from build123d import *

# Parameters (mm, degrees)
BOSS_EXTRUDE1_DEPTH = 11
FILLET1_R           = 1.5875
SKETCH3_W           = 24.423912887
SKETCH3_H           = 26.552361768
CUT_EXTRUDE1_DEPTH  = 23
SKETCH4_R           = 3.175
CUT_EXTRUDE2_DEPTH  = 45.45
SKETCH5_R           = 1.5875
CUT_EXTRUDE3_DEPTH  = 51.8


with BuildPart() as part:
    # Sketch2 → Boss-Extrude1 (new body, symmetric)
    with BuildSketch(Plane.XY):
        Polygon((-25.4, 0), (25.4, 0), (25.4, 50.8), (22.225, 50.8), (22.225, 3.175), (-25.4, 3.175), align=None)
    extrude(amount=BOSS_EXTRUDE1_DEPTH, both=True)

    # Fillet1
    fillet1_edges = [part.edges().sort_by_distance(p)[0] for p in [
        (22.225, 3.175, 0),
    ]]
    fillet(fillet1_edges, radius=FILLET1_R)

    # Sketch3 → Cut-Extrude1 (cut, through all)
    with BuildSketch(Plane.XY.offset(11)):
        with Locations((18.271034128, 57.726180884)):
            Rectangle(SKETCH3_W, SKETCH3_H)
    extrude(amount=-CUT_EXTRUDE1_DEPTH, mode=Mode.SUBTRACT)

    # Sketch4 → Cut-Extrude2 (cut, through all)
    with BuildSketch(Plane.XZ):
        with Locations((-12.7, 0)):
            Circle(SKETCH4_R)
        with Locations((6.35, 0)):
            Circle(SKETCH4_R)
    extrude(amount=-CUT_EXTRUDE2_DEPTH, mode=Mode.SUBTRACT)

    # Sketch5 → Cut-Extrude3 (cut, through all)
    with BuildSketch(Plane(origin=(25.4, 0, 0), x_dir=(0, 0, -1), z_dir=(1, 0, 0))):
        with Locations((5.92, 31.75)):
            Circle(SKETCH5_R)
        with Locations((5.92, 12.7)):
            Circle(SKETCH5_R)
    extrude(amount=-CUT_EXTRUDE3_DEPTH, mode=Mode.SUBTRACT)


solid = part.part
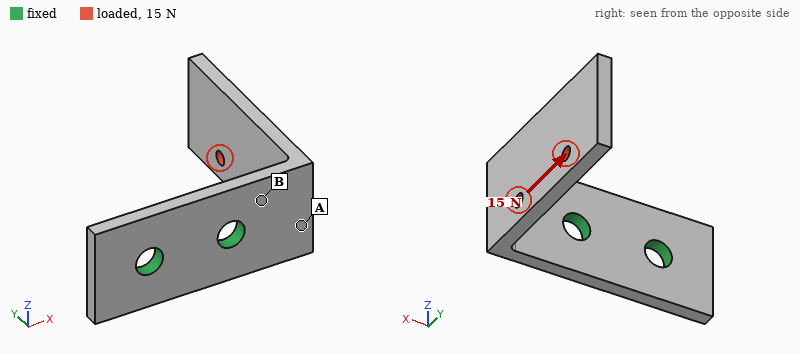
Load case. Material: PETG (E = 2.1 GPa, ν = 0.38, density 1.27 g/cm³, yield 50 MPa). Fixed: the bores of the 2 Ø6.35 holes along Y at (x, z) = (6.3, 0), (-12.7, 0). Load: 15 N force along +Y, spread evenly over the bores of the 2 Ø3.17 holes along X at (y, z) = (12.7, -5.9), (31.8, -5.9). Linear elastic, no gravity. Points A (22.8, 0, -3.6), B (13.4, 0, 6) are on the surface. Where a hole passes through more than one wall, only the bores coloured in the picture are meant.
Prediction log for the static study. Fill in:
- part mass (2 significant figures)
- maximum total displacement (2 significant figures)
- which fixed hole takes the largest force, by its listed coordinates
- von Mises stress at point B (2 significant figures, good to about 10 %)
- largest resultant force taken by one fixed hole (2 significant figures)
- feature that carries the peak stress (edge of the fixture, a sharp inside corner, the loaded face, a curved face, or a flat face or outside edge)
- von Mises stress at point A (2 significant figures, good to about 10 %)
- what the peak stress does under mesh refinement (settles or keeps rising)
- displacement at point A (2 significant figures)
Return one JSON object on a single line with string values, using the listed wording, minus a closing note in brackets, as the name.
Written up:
{"part mass": "7.9 g", "maximum total displacement": "0.72 mm", "which fixed hole takes the largest force, by its listed coordinates": "(6.3, 0)", "von Mises stress at point B": "3.6 MPa", "largest resultant force taken by one fixed hole": "16 N", "feature that carries the peak stress": "edge of the fixture", "von Mises stress at point A": "1.1 MPa", "what the peak stress does under mesh refinement": "keeps rising", "displacement at point A": "0.17 mm"}
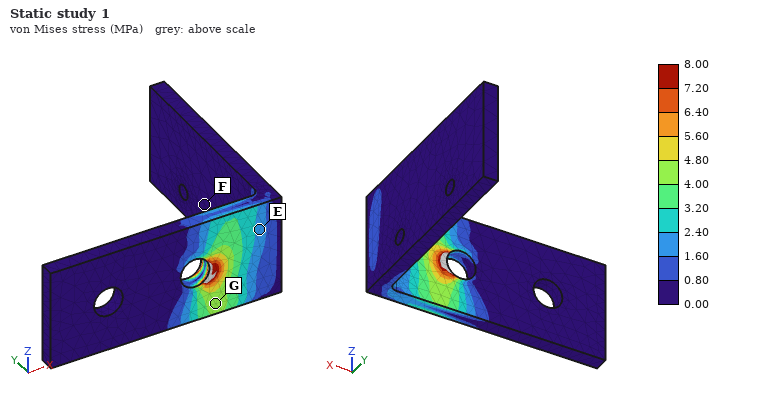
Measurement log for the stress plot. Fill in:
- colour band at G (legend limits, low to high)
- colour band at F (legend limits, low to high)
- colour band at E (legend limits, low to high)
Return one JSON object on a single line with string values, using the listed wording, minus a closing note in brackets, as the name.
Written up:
{"colour band at G": "4.00 to 4.80 MPa", "colour band at F": "0.00 to 0.80 MPa", "colour band at E": "1.60 to 2.40 MPa"}
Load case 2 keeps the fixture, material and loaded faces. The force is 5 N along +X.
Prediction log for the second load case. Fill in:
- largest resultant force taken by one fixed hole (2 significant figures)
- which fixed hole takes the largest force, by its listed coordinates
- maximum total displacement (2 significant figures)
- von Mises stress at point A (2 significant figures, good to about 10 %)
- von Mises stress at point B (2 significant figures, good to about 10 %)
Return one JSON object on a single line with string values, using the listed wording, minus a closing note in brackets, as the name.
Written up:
{"largest resultant force taken by one fixed hole": "4.5 N", "which fixed hole takes the largest force, by its listed coordinates": "(6.3, 0)", "maximum total displacement": "0.84 mm", "von Mises stress at point A": "1.5 MPa", "von Mises stress at point B": "2.4 MPa"}
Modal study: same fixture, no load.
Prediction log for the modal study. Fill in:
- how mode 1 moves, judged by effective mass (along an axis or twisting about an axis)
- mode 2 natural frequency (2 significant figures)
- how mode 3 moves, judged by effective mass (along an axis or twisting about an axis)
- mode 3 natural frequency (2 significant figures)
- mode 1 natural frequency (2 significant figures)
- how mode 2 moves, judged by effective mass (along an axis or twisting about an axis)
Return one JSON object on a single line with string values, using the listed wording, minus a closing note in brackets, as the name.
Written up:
{"how mode 1 moves, judged by effective mass": "along X", "mode 2 natural frequency": "390 Hz", "how mode 3 moves, judged by effective mass": "along Y", "mode 3 natural frequency": "1000 Hz", "mode 1 natural frequency": "240 Hz", "how mode 2 moves, judged by effective mass": "along Z"}
